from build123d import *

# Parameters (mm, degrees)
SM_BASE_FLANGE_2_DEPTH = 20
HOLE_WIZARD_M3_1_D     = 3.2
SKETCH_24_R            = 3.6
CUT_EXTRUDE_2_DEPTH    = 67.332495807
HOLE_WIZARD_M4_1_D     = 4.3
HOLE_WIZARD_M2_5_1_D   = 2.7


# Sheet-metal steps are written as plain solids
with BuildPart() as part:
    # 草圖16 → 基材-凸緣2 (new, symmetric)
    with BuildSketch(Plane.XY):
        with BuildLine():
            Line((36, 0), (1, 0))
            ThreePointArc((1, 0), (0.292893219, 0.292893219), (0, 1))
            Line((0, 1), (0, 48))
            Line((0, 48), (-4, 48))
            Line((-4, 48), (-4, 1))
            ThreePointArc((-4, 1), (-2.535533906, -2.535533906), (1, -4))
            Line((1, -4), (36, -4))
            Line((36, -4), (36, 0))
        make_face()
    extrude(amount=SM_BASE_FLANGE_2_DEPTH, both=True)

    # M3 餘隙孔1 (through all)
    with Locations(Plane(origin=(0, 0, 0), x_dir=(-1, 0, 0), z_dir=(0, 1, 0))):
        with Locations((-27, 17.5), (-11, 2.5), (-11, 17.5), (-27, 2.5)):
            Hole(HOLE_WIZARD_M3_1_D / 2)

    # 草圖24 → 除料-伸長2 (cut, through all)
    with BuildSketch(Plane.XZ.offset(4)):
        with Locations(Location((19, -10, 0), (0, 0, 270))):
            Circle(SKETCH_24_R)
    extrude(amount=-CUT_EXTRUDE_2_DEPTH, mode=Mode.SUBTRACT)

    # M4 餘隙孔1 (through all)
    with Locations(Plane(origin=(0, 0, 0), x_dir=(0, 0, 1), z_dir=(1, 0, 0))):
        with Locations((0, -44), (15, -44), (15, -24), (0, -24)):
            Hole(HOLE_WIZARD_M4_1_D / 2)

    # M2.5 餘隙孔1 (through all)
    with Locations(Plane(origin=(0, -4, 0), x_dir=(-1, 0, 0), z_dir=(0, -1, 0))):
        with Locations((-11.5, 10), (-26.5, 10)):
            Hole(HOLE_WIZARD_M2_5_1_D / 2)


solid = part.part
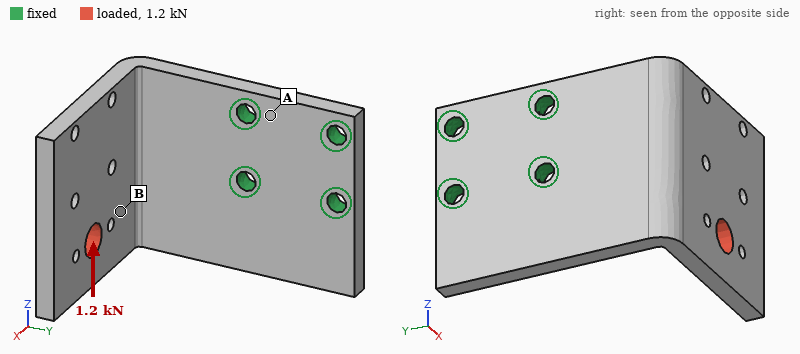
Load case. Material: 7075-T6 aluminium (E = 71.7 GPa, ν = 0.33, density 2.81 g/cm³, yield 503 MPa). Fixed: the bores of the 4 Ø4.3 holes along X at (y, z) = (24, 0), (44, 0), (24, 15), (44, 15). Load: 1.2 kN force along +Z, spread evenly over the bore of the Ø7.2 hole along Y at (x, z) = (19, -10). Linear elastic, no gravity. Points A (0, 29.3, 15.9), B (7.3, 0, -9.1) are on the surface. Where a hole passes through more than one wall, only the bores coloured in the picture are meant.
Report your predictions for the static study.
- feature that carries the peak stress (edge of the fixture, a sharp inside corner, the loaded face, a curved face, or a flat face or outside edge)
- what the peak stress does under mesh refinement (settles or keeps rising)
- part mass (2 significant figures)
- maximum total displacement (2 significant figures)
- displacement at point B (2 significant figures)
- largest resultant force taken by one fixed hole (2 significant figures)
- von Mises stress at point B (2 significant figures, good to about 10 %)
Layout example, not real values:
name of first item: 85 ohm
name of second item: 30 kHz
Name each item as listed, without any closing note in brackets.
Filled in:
feature that carries the peak stress: edge of the fixture
what the peak stress does under mesh refinement: keeps rising
part mass: 37 g
maximum total displacement: 0.88 mm
displacement at point B: 0.30 mm
largest resultant force taken by one fixed hole: 1.9 kN
von Mises stress at point B: 75 MPa
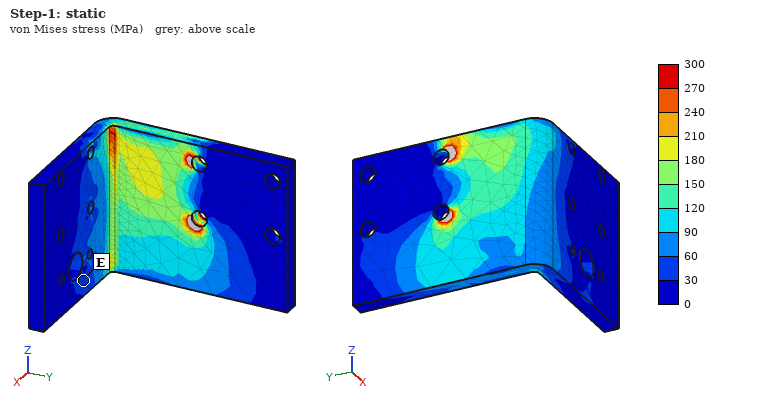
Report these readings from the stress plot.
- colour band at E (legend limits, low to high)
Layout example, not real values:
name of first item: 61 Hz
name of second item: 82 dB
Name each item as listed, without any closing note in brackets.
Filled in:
colour band at E: 30 to 60 MPa
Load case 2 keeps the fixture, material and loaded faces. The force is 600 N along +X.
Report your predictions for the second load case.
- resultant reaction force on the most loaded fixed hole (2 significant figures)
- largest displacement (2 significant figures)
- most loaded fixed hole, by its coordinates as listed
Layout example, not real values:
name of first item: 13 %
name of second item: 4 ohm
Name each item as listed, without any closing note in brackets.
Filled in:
resultant reaction force on the most loaded fixed hole: 990 N
largest displacement: 0.71 mm
most loaded fixed hole, by its coordinates as listed: (24, 0)
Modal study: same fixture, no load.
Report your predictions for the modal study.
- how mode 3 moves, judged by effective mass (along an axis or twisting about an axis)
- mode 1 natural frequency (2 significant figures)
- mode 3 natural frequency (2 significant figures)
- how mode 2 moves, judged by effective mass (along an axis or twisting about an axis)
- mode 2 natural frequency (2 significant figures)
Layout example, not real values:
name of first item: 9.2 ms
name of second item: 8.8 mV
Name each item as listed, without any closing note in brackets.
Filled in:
how mode 3 moves, judged by effective mass: along X
mode 1 natural frequency: 1100 Hz
mode 3 natural frequency: 3100 Hz
how mode 2 moves, judged by effective mass: along Z
mode 2 natural frequency: 1800 Hz
